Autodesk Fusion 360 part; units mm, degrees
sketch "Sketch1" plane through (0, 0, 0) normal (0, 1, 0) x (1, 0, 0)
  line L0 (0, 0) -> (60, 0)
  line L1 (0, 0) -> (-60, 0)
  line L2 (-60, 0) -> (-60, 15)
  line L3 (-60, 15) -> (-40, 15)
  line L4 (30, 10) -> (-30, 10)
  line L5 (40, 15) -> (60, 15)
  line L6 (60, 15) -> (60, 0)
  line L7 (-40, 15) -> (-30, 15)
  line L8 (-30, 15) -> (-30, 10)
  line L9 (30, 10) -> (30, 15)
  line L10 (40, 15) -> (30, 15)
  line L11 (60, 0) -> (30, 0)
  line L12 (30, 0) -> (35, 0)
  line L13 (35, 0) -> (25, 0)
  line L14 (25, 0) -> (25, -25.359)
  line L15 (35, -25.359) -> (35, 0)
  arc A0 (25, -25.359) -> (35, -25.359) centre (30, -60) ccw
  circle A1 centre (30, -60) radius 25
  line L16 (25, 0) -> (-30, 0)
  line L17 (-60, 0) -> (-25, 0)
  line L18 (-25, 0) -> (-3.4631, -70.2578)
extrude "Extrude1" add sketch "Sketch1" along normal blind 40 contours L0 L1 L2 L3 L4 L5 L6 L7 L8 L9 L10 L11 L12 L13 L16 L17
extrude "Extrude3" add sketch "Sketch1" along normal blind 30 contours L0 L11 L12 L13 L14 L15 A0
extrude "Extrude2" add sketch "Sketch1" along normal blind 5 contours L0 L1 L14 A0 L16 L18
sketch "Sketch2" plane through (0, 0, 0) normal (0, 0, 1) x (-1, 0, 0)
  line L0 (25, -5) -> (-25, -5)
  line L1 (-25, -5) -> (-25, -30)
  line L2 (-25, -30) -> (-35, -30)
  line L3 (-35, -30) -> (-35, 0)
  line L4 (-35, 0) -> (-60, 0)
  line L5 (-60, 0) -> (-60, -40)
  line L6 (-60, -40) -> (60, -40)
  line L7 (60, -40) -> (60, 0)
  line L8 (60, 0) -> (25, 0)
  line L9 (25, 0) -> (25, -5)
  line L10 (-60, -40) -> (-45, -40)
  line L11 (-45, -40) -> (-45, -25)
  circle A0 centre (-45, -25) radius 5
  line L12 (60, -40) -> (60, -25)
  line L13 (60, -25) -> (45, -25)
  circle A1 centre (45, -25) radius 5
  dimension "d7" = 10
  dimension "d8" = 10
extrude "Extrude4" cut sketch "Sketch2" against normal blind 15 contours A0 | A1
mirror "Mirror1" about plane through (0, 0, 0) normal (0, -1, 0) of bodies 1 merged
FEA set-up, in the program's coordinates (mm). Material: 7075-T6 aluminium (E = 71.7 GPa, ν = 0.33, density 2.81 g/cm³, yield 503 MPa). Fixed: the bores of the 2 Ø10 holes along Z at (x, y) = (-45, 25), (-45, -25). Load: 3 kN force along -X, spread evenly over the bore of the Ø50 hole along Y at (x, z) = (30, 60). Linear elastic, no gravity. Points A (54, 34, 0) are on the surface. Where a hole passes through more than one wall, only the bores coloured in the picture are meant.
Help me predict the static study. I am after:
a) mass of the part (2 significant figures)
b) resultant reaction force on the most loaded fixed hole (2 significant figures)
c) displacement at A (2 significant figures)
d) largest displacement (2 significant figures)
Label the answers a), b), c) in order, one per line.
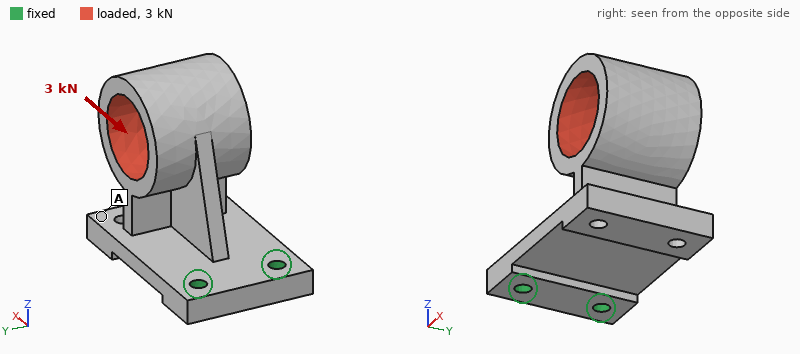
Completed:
a) 730 g
b) 1.7 kN
c) 0.80 mm
d) 1.2 mm
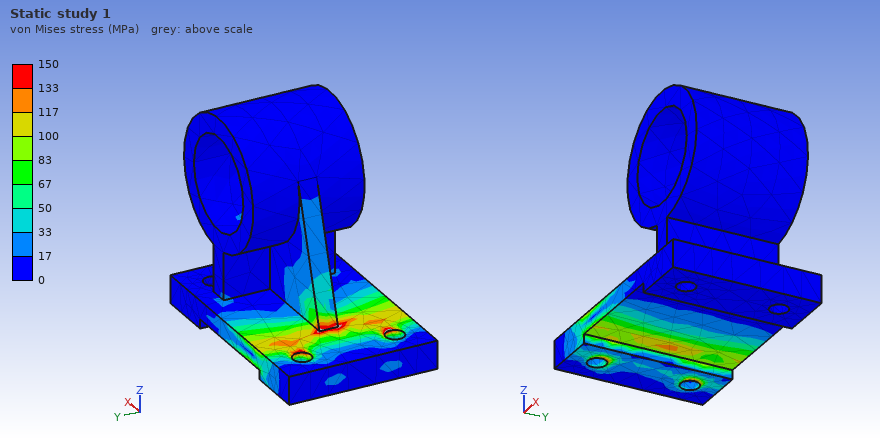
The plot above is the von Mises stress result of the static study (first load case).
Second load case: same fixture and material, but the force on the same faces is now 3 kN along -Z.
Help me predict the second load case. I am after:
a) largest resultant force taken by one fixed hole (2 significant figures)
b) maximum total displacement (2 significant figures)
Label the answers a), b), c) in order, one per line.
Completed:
a) 1.5 kN
b) 1.1 mm
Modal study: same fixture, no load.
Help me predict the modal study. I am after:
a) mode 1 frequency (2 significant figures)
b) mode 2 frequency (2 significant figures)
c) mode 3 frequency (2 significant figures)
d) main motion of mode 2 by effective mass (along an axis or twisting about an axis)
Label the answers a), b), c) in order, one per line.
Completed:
a) 380 Hz
b) 590 Hz
c) 2300 Hz
d) along Y
